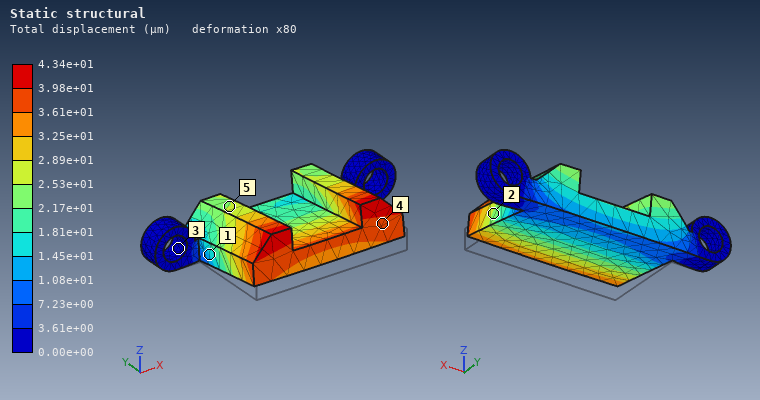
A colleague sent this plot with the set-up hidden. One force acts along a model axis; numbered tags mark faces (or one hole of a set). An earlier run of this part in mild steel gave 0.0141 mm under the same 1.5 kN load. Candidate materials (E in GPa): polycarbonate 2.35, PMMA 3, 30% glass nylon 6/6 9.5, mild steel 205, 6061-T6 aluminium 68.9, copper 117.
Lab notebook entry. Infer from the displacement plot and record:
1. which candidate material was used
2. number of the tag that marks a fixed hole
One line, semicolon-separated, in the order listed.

6061-T6 aluminium; 3
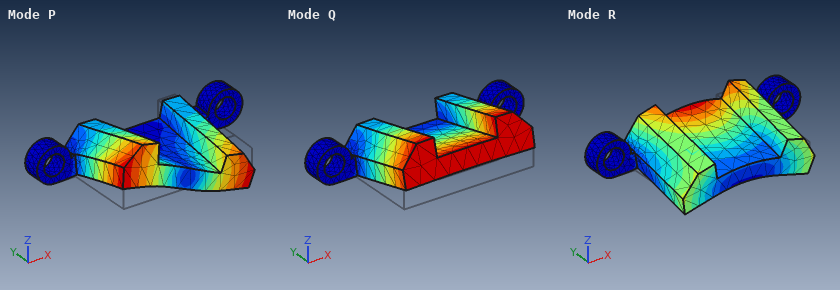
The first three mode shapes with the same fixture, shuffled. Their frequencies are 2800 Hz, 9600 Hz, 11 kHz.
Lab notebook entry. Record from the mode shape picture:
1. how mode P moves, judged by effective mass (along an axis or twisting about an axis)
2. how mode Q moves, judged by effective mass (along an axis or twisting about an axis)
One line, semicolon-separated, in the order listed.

twisting about Y; along Z
